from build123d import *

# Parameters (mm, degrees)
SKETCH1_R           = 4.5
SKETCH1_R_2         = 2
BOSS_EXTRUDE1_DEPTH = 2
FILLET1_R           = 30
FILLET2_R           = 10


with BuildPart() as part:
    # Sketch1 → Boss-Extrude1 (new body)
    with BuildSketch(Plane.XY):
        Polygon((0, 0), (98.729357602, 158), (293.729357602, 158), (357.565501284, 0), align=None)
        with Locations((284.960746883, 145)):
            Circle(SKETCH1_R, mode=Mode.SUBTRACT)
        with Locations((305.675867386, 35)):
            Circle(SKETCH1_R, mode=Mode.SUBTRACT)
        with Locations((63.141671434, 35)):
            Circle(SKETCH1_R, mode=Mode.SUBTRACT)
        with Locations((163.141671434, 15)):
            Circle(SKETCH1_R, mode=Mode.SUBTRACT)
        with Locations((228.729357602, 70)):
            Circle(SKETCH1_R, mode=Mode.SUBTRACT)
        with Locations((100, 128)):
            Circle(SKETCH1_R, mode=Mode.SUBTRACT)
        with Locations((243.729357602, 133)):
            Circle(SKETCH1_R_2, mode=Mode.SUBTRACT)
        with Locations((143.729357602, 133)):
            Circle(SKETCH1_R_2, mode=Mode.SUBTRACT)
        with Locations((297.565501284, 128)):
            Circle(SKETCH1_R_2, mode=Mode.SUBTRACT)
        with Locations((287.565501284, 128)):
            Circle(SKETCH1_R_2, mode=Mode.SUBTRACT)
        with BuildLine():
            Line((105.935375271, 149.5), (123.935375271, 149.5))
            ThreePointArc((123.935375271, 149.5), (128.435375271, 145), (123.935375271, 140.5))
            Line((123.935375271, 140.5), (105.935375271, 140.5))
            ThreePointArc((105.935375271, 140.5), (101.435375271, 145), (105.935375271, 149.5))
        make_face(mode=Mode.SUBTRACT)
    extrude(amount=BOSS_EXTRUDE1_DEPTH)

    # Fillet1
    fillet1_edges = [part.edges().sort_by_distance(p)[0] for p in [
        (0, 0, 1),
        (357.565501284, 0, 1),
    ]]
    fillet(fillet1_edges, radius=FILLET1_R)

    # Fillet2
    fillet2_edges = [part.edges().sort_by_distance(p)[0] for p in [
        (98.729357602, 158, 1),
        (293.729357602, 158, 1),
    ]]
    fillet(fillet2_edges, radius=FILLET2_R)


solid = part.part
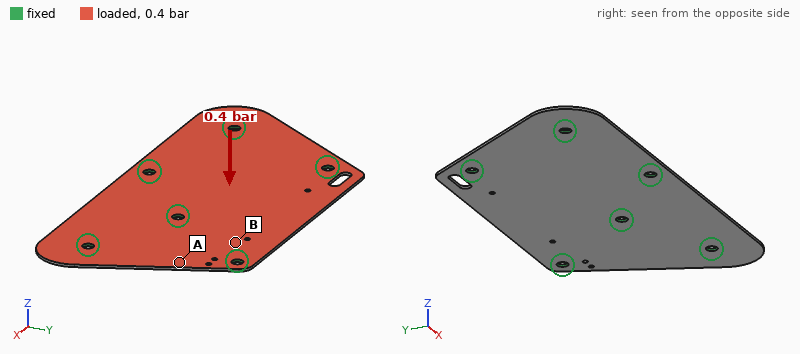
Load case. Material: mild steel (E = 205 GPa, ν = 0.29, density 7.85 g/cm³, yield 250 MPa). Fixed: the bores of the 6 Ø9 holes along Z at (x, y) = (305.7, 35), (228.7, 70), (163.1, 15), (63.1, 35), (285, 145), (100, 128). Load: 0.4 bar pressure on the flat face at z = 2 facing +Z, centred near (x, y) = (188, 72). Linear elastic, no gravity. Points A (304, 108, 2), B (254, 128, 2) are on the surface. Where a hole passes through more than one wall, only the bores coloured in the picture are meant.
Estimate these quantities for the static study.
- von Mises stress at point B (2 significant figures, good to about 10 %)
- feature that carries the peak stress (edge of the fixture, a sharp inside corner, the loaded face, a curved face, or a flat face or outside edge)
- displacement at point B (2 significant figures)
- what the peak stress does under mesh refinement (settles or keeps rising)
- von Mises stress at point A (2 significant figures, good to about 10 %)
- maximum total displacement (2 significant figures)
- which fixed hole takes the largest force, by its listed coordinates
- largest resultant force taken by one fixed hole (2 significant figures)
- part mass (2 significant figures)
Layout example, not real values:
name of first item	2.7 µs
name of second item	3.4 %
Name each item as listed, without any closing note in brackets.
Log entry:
von Mises stress at point B	51 MPa
feature that carries the peak stress	edge of the fixture
displacement at point B	0.14 mm
what the peak stress does under mesh refinement	keeps rising
von Mises stress at point A	18 MPa
maximum total displacement	0.69 mm
which fixed hole takes the largest force, by its listed coordinates	(228.7, 70)
largest resultant force taken by one fixed hole	410 N
part mass	660 g
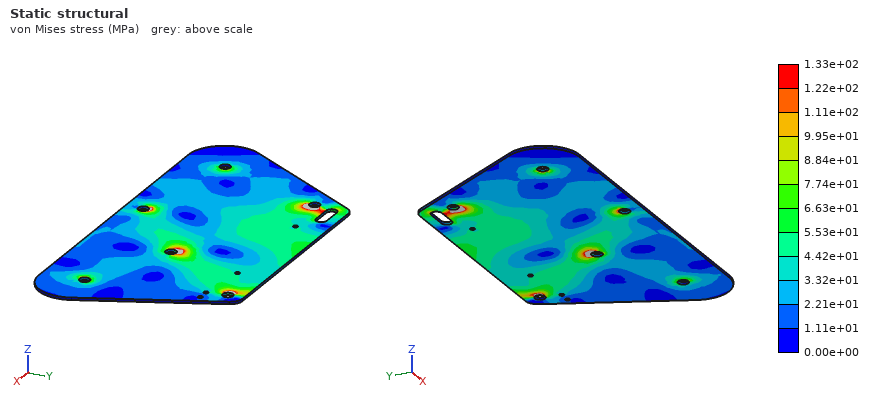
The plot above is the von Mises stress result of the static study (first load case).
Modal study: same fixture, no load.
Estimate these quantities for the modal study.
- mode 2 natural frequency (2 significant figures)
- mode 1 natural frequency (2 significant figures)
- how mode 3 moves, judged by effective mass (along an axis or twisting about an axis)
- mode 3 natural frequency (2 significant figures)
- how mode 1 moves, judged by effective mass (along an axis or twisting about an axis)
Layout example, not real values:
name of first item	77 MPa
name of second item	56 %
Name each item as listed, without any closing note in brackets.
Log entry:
mode 2 natural frequency	690 Hz
mode 1 natural frequency	410 Hz
how mode 3 moves, judged by effective mass	along Z
mode 3 natural frequency	750 Hz
how mode 1 moves, judged by effective mass	along Z
